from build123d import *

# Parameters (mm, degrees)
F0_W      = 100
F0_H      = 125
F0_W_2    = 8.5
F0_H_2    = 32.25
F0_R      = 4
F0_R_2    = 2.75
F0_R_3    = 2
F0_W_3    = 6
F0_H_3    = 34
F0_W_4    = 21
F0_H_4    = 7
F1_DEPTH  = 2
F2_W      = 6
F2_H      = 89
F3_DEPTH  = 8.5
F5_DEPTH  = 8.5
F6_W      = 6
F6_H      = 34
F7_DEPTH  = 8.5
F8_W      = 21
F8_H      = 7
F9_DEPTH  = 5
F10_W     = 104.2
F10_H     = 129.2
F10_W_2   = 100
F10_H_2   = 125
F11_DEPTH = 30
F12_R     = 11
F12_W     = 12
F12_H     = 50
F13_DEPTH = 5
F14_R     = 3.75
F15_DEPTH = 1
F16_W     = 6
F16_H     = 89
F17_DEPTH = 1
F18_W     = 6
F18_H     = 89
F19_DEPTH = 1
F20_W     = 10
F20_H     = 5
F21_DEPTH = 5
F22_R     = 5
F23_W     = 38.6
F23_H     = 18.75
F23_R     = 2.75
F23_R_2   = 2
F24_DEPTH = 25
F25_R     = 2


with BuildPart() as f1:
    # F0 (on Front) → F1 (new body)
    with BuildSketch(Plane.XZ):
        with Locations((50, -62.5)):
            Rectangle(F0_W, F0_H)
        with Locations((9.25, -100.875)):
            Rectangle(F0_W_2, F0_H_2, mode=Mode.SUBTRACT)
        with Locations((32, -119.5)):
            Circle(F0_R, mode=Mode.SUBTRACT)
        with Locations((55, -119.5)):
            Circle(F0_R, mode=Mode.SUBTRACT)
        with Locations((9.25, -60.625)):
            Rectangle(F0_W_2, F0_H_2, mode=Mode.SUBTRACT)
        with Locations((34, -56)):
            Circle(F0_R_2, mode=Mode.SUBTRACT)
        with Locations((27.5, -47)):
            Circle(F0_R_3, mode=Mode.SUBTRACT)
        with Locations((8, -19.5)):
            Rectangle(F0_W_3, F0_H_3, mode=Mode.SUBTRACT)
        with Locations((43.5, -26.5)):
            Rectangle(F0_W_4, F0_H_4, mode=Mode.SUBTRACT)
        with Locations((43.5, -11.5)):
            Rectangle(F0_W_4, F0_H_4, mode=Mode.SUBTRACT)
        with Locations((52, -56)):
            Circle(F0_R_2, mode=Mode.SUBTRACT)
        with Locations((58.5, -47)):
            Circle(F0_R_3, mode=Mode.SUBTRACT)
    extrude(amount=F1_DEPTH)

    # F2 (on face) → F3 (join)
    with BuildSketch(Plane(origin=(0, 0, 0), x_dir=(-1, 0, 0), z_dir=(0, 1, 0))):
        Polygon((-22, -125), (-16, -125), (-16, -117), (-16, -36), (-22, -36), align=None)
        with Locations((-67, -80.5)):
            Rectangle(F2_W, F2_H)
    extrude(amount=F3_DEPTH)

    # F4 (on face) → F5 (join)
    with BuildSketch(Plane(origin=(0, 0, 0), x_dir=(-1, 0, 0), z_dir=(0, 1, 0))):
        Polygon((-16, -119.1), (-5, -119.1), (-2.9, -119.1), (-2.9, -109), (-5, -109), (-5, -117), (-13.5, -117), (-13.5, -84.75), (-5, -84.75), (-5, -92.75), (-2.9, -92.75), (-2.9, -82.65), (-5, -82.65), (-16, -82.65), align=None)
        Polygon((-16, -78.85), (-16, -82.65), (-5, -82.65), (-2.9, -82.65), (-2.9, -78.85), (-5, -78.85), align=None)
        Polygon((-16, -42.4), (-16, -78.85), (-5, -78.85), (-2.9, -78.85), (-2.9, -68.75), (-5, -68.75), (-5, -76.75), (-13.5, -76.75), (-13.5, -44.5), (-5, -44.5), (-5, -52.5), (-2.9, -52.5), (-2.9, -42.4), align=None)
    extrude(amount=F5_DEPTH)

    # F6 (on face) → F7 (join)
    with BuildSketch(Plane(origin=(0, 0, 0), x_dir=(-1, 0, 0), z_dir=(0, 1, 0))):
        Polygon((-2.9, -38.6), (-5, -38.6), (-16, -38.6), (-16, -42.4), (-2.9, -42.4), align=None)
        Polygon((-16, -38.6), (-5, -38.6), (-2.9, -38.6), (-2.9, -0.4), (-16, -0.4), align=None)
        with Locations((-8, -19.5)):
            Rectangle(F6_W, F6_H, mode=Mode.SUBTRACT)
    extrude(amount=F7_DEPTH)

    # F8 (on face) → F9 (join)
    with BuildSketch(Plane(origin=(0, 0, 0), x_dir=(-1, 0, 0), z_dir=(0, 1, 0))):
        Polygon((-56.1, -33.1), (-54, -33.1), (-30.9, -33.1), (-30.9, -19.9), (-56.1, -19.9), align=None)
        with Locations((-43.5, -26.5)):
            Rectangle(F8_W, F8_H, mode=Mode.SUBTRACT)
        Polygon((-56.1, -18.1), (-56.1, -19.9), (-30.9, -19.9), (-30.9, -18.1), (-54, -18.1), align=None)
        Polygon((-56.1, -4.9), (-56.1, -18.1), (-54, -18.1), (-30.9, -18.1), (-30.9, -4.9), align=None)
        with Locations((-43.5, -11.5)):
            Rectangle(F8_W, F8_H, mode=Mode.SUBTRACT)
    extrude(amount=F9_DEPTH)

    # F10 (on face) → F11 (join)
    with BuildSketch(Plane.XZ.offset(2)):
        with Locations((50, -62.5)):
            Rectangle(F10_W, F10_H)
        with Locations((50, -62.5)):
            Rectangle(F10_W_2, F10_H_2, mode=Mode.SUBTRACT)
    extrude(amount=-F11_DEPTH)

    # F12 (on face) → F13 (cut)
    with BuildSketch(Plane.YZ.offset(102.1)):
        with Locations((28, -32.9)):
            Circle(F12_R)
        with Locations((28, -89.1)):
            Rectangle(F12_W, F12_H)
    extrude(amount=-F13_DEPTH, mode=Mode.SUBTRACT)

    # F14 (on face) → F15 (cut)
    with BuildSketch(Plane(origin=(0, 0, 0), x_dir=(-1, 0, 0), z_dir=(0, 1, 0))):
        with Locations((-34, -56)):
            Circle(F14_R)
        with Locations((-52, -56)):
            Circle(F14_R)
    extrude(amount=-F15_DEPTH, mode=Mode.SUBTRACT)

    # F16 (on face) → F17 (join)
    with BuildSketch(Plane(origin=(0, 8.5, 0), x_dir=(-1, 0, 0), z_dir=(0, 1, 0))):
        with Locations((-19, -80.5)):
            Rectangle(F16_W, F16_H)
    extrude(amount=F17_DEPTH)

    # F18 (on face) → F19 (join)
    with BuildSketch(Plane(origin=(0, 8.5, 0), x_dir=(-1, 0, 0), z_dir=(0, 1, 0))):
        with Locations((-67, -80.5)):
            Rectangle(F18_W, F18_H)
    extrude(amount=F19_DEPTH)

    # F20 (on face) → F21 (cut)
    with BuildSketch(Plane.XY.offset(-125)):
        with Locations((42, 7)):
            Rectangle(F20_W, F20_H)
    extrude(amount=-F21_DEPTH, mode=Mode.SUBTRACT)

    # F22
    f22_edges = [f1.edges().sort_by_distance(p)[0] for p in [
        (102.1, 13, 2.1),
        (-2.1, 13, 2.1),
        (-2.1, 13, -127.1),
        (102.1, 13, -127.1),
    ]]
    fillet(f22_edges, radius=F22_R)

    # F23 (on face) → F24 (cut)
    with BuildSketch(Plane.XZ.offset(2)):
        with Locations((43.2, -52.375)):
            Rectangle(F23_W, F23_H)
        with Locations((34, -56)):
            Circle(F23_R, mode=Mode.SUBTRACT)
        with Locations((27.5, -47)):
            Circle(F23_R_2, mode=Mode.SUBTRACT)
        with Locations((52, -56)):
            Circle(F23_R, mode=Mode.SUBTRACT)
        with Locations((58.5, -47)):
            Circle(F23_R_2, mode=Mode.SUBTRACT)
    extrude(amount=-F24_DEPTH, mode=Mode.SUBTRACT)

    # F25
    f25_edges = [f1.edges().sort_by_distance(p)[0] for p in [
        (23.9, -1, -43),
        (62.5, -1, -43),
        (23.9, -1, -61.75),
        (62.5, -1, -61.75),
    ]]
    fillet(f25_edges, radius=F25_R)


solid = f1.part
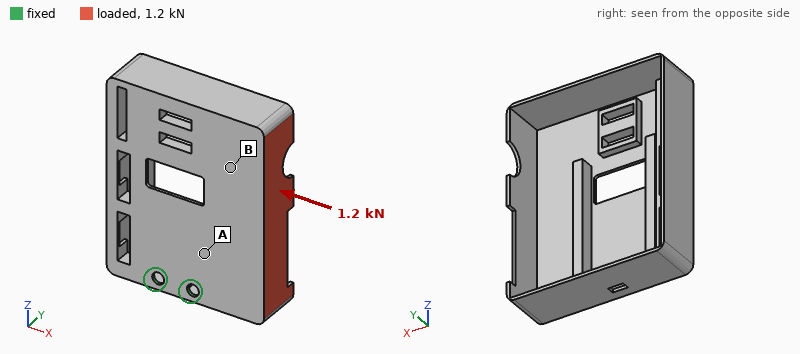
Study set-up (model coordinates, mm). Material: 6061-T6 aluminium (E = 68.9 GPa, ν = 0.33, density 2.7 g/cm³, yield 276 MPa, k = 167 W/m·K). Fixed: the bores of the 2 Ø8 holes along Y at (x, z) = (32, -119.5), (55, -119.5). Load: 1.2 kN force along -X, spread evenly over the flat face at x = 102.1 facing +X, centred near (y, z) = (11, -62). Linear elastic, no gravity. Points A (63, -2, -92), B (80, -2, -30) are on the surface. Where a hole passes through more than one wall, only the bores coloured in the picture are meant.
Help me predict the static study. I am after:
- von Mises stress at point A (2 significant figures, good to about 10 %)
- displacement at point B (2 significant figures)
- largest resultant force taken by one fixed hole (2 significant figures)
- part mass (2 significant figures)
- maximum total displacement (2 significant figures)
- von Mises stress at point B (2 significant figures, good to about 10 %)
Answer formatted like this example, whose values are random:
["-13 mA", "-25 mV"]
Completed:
["20 MPa", "0.51 mm", "2.3 kN", "180 g", "1.7 mm", "43 MPa"]
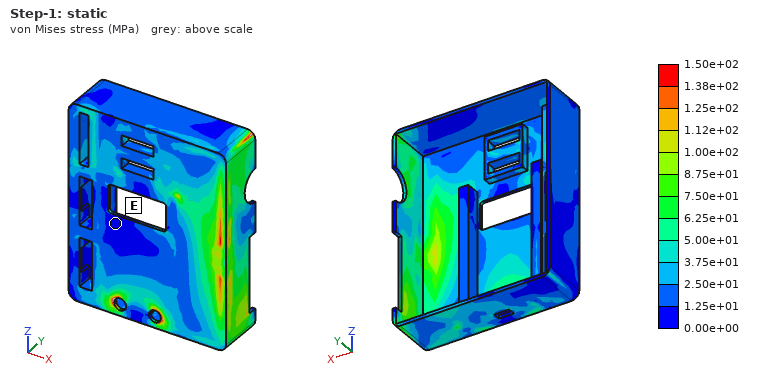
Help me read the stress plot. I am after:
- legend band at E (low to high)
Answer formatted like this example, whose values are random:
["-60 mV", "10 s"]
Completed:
["0.00e+00 to 1.25e+01 MPa"]
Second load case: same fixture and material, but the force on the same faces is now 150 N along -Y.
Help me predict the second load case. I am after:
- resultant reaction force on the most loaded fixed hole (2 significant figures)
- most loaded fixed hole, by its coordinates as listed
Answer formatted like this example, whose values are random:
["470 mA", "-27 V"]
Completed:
["340 N", "(55, -119.5)"]
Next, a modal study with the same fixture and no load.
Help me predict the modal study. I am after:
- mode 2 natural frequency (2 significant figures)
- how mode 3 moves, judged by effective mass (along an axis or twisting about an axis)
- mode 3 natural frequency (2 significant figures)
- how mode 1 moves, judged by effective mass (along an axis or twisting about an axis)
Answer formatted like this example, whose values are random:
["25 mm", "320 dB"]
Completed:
["360 Hz", "along X", "1100 Hz", "along Y"]
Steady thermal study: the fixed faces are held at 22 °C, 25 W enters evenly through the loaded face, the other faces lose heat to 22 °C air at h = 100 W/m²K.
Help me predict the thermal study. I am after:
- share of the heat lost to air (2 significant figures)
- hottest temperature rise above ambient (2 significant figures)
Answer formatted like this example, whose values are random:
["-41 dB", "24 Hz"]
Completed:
["84 %", "19 K"]
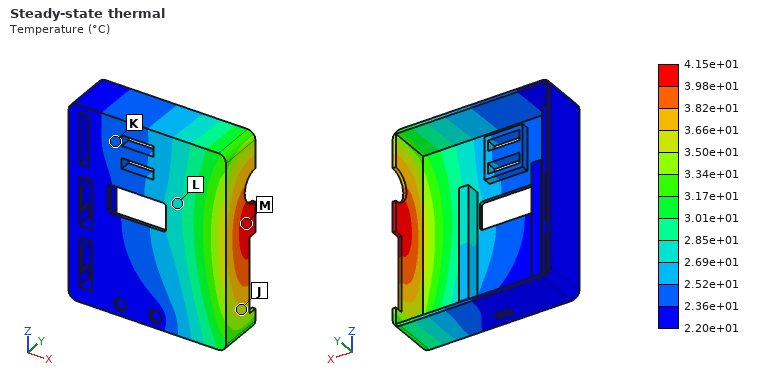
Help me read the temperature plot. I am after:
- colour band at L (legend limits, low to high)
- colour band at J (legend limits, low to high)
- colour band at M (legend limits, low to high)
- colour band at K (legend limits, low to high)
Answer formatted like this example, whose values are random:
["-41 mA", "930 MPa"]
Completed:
["2.69e+01 to 2.85e+01 °C", "3.50e+01 to 3.66e+01 °C", "3.98e+01 to 4.15e+01 °C", "2.36e+01 to 2.52e+01 °C"]
